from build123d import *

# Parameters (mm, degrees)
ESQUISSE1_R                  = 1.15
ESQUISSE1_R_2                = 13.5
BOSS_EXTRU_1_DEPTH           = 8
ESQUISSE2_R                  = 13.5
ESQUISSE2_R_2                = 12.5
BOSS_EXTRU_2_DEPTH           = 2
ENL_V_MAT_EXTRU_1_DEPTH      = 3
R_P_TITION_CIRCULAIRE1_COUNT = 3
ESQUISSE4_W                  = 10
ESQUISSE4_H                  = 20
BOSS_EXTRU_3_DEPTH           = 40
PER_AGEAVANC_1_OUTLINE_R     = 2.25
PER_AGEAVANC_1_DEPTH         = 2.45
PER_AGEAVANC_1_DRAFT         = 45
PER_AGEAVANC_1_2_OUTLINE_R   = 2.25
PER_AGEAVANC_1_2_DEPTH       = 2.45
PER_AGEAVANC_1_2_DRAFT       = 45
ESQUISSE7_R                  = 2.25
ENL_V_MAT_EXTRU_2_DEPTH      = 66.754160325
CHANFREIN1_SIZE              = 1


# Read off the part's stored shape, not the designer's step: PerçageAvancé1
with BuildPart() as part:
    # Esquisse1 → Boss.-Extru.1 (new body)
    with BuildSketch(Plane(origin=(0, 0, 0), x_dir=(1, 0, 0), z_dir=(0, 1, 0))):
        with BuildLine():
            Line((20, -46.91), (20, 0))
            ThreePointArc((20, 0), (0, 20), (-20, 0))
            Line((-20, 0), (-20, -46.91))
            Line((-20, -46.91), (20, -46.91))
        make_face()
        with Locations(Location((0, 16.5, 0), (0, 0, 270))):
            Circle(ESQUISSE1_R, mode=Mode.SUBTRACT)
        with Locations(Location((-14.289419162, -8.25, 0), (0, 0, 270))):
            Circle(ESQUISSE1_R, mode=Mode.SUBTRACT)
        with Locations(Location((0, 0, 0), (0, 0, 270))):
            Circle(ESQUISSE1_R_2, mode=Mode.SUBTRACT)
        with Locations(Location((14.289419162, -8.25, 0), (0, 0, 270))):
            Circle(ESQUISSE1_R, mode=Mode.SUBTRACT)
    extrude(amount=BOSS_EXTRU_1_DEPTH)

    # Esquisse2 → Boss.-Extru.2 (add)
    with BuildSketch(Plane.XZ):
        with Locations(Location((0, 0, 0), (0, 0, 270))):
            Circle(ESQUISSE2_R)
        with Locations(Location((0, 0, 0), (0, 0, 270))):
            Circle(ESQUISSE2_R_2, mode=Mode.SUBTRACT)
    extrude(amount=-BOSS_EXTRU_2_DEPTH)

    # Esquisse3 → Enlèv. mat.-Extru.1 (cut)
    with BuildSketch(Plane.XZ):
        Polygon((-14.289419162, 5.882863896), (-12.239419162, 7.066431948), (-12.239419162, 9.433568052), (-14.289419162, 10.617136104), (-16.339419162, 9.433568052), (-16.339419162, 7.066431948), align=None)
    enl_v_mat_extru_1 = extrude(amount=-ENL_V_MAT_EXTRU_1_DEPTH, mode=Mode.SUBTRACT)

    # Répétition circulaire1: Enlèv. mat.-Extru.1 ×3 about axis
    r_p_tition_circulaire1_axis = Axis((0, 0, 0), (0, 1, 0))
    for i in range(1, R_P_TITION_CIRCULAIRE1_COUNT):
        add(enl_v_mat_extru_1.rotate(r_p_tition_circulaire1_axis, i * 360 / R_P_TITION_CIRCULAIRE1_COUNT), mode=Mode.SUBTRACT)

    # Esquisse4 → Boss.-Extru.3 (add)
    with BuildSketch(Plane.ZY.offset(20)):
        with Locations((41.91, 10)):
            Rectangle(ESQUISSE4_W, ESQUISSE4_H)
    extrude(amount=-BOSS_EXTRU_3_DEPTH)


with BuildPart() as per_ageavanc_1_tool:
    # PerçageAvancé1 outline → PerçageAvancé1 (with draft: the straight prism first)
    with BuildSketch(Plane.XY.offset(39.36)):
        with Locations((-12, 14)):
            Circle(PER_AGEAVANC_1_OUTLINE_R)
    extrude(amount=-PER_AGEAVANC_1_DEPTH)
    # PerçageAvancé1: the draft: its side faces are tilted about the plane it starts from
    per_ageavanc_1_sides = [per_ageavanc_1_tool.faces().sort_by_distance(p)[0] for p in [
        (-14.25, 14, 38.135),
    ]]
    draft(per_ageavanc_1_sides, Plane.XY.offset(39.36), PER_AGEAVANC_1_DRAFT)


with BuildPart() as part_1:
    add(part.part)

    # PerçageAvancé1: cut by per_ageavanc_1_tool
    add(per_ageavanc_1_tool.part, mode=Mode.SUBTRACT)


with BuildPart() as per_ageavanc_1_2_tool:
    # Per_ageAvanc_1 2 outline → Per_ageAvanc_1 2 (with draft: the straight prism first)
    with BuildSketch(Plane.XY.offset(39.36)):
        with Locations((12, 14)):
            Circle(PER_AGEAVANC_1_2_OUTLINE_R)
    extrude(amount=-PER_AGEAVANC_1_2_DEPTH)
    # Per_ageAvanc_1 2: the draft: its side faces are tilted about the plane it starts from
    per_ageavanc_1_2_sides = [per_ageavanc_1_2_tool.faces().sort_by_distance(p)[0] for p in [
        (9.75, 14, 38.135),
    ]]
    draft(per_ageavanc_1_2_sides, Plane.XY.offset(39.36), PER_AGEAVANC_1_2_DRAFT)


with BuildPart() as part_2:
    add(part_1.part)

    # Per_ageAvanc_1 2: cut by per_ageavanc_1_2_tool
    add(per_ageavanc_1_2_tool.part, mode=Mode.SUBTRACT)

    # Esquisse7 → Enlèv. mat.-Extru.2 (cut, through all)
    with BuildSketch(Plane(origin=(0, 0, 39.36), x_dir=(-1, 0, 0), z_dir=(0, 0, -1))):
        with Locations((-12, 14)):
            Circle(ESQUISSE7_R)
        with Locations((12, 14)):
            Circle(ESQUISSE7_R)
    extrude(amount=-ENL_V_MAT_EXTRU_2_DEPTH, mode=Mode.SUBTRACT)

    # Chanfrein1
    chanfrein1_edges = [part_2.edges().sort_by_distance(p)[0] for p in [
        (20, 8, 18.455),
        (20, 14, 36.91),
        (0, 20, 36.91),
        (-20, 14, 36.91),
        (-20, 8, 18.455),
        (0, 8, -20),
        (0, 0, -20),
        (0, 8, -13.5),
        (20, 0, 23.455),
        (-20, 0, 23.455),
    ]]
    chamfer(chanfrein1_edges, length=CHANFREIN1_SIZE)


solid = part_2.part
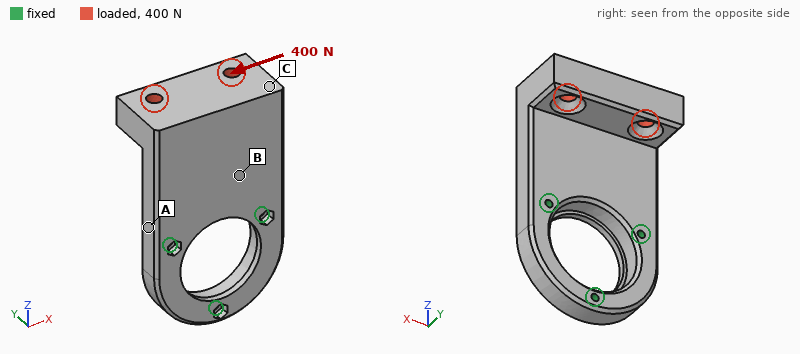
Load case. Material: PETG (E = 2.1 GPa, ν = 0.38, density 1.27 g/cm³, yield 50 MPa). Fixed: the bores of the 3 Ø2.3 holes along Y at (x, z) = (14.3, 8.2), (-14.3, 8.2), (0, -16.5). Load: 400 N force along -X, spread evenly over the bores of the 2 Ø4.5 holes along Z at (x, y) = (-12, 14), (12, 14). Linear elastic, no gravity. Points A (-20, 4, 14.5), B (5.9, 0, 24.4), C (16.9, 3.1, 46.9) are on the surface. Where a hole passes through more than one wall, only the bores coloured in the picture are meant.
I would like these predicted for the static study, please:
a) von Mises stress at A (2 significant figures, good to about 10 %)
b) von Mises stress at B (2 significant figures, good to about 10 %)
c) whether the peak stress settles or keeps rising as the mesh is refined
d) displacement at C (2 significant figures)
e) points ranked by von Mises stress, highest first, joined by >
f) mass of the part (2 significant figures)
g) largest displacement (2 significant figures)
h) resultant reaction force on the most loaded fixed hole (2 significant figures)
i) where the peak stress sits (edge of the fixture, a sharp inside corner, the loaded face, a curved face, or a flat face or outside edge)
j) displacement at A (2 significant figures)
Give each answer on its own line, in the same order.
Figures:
9.1 MPa
4.6 MPa
keeps rising
0.44 mm
A > B > C
25 g
0.73 mm
480 N
edge of the fixture
0.12 mm
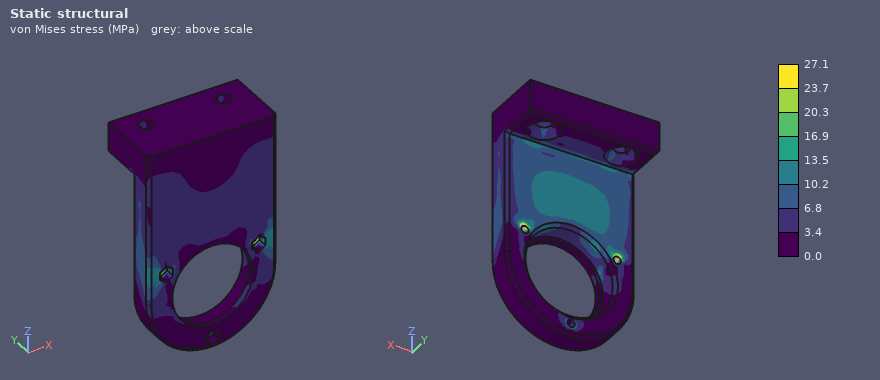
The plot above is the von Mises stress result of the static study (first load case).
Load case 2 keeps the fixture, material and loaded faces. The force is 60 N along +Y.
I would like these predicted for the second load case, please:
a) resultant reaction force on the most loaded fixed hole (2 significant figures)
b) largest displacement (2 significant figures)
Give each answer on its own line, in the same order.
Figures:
43 N
0.77 mm
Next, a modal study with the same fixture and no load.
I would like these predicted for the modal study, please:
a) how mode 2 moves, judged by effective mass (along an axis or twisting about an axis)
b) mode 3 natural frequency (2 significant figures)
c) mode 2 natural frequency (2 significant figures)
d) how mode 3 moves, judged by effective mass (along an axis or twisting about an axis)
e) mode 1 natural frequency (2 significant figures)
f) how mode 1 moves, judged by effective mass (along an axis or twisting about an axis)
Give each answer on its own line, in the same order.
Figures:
along X
2300 Hz
1300 Hz
along X
460 Hz
along Y
